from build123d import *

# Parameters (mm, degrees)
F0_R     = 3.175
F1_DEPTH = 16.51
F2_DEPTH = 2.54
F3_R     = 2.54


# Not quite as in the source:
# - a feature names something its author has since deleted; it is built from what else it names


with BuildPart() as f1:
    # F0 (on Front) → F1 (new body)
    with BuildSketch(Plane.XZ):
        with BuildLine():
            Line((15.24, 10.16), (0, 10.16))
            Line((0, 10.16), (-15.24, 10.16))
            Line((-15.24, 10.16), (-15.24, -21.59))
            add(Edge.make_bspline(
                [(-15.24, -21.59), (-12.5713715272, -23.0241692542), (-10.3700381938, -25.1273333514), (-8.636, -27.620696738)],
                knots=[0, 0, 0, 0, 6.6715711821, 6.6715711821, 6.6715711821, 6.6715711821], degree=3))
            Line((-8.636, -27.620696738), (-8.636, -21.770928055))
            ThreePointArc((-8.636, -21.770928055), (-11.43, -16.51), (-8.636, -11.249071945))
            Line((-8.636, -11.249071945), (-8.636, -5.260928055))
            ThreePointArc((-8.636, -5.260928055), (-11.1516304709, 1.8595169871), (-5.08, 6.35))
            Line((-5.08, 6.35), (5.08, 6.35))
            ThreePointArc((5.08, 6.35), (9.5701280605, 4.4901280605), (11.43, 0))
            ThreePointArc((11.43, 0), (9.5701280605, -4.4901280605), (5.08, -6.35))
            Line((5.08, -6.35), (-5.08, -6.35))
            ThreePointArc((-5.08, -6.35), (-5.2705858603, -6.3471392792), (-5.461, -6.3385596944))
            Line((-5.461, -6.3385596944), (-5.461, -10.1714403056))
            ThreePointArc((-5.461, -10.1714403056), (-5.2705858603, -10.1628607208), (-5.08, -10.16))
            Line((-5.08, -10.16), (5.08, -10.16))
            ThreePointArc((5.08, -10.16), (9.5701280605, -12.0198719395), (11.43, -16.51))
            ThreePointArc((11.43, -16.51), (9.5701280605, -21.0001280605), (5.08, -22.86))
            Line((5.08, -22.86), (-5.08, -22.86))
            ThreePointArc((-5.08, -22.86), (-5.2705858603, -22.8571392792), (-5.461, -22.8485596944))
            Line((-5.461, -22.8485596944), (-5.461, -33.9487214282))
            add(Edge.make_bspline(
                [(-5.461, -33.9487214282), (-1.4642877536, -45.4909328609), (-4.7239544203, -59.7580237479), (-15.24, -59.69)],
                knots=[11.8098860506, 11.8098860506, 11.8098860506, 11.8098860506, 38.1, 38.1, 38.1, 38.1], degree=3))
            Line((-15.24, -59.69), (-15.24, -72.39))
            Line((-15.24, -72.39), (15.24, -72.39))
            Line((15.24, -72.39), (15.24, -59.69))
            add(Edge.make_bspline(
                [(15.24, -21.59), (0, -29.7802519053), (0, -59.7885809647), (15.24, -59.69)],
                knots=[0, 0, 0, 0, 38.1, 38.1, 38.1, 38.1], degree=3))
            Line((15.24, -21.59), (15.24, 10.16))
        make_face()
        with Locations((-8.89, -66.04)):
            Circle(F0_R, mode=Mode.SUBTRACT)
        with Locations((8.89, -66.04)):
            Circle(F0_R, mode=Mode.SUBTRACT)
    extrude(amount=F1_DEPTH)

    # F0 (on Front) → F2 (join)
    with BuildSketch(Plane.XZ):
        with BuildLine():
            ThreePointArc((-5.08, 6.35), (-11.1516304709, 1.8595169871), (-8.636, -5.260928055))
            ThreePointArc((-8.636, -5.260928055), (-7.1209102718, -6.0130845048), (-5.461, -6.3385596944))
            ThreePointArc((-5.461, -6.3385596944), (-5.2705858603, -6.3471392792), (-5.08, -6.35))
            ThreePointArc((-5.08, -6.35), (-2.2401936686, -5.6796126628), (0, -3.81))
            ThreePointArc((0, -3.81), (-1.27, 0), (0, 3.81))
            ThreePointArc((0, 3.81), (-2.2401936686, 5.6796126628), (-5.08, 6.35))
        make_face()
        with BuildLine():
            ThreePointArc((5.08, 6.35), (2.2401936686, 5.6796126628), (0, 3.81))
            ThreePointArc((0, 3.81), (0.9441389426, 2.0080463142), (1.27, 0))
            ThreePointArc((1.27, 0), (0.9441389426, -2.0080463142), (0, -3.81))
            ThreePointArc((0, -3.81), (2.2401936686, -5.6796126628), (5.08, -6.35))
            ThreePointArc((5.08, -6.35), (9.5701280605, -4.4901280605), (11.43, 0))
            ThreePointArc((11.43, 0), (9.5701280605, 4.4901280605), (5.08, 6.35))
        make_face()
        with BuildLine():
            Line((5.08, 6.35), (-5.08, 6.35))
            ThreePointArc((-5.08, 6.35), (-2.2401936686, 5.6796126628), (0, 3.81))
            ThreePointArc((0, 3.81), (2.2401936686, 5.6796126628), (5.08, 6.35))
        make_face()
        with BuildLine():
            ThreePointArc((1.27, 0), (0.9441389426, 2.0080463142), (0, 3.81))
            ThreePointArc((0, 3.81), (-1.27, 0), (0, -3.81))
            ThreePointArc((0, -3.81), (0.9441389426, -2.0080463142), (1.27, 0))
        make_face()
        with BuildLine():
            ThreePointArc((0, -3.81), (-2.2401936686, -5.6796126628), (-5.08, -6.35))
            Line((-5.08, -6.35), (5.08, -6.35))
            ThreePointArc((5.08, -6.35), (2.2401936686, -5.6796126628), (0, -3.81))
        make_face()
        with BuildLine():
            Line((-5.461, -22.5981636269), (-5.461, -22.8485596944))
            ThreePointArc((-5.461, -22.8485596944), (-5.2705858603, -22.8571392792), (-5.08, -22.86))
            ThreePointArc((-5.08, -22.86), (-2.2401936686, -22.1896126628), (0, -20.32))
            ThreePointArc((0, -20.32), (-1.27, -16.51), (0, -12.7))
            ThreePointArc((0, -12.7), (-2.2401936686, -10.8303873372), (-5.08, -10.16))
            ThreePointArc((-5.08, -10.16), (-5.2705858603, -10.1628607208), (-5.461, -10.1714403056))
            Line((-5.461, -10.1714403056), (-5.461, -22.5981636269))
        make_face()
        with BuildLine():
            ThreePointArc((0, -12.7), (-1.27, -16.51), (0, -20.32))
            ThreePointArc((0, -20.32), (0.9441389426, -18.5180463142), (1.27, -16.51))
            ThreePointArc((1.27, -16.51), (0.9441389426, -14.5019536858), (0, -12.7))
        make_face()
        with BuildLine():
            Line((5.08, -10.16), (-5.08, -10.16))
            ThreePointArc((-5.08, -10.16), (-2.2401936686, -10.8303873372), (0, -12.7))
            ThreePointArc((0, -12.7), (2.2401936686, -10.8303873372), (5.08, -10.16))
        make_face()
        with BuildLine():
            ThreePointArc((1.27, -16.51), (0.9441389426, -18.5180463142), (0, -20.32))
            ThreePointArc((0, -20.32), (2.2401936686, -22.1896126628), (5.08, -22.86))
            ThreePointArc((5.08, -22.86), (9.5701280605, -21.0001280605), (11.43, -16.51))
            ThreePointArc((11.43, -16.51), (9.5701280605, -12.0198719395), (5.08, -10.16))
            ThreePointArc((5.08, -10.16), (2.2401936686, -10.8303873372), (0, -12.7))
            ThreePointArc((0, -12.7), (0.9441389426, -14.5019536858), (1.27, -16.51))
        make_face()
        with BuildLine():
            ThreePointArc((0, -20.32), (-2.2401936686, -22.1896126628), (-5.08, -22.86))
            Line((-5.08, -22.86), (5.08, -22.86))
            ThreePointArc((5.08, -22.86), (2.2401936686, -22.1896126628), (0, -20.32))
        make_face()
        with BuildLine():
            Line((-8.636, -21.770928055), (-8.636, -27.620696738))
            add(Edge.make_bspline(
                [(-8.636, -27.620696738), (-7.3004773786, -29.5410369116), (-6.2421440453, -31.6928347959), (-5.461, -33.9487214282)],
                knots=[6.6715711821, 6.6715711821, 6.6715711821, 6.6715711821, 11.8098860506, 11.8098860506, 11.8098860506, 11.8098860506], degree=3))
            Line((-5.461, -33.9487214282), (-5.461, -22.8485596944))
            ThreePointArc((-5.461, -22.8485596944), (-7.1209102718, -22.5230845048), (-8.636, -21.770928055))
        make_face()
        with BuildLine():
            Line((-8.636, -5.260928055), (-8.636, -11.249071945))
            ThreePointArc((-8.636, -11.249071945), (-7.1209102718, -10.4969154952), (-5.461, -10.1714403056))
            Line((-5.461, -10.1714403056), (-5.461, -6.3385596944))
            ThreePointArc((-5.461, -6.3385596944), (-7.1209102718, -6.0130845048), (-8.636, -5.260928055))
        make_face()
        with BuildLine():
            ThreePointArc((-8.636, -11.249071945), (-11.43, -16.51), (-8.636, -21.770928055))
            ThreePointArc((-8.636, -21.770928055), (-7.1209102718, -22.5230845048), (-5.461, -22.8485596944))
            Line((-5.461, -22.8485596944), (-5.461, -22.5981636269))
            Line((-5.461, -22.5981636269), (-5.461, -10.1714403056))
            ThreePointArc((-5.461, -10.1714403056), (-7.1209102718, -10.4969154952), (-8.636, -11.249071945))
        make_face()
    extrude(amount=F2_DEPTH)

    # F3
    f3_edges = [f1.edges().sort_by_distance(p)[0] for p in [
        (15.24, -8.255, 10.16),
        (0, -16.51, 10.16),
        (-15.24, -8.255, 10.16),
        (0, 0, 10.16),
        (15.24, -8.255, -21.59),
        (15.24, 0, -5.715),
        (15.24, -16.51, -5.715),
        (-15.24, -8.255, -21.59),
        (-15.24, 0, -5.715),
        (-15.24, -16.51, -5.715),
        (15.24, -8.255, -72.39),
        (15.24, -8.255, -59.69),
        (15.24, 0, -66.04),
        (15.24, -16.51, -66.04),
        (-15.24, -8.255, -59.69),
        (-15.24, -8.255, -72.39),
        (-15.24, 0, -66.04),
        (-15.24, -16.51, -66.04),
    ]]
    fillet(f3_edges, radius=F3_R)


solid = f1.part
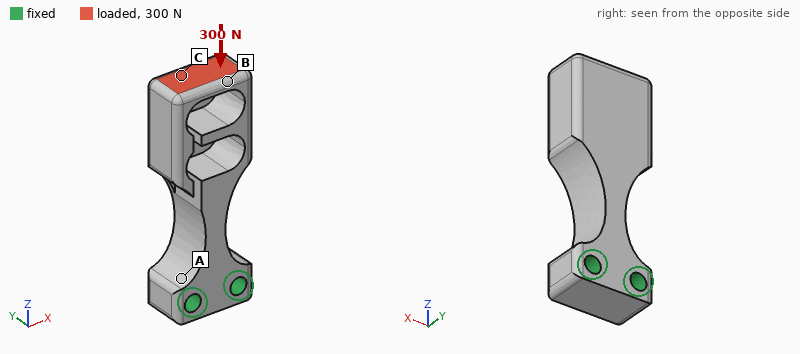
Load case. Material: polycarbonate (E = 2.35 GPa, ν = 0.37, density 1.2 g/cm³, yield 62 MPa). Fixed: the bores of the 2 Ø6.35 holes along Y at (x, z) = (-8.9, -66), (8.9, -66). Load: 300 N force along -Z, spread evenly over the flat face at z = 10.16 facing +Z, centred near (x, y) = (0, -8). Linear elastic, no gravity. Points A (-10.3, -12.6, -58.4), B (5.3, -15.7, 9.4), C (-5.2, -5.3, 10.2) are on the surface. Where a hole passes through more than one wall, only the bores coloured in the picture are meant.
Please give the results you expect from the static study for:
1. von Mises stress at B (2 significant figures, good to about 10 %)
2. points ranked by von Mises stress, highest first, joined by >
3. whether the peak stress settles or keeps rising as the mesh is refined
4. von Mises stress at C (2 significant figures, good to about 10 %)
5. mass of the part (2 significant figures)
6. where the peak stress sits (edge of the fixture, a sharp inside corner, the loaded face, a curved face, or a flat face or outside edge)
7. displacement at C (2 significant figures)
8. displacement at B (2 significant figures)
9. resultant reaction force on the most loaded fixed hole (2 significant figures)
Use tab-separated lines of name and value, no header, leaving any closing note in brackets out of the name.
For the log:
von Mises stress at B	5.2 MPa
points ranked by von Mises stress, highest first, joined by >	B > C > A
whether the peak stress settles or keeps rising as the mesh is refined	keeps rising
von Mises stress at C	3.1 MPa
mass of the part	26 g
where the peak stress sits	a sharp inside corner
displacement at C	0.80 mm
displacement at B	0.66 mm
resultant reaction force on the most loaded fixed hole	160 N
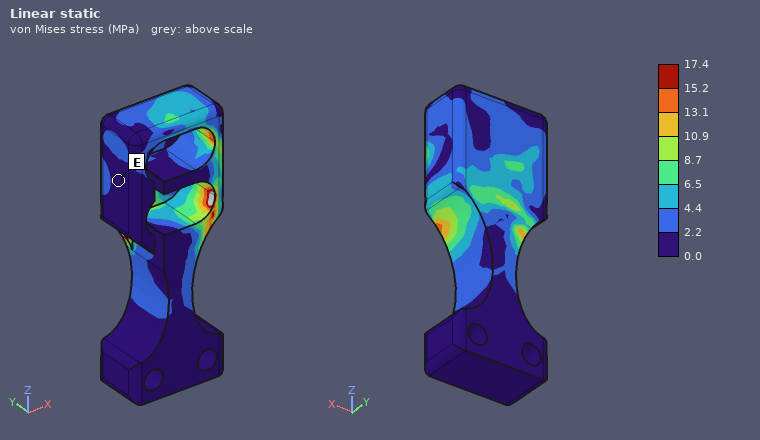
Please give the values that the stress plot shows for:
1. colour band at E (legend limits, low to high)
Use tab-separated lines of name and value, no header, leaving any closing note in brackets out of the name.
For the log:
colour band at E	0.0 to 2.2 MPa
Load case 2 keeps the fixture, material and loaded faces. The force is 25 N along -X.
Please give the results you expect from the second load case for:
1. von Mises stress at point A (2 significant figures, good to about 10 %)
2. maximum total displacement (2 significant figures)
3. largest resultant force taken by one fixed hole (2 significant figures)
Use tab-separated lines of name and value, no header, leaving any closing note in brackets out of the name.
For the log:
von Mises stress at point A	0.65 MPa
maximum total displacement	1.0 mm
largest resultant force taken by one fixed hole	110 N
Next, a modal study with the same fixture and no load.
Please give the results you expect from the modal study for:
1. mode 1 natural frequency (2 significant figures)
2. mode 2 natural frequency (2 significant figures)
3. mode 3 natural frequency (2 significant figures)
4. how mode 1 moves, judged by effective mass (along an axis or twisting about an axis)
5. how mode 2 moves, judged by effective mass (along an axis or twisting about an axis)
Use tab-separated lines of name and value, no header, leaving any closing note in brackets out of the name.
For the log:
mode 1 natural frequency	310 Hz
mode 2 natural frequency	410 Hz
mode 3 natural frequency	920 Hz
how mode 1 moves, judged by effective mass	along X
how mode 2 moves, judged by effective mass	along Y
